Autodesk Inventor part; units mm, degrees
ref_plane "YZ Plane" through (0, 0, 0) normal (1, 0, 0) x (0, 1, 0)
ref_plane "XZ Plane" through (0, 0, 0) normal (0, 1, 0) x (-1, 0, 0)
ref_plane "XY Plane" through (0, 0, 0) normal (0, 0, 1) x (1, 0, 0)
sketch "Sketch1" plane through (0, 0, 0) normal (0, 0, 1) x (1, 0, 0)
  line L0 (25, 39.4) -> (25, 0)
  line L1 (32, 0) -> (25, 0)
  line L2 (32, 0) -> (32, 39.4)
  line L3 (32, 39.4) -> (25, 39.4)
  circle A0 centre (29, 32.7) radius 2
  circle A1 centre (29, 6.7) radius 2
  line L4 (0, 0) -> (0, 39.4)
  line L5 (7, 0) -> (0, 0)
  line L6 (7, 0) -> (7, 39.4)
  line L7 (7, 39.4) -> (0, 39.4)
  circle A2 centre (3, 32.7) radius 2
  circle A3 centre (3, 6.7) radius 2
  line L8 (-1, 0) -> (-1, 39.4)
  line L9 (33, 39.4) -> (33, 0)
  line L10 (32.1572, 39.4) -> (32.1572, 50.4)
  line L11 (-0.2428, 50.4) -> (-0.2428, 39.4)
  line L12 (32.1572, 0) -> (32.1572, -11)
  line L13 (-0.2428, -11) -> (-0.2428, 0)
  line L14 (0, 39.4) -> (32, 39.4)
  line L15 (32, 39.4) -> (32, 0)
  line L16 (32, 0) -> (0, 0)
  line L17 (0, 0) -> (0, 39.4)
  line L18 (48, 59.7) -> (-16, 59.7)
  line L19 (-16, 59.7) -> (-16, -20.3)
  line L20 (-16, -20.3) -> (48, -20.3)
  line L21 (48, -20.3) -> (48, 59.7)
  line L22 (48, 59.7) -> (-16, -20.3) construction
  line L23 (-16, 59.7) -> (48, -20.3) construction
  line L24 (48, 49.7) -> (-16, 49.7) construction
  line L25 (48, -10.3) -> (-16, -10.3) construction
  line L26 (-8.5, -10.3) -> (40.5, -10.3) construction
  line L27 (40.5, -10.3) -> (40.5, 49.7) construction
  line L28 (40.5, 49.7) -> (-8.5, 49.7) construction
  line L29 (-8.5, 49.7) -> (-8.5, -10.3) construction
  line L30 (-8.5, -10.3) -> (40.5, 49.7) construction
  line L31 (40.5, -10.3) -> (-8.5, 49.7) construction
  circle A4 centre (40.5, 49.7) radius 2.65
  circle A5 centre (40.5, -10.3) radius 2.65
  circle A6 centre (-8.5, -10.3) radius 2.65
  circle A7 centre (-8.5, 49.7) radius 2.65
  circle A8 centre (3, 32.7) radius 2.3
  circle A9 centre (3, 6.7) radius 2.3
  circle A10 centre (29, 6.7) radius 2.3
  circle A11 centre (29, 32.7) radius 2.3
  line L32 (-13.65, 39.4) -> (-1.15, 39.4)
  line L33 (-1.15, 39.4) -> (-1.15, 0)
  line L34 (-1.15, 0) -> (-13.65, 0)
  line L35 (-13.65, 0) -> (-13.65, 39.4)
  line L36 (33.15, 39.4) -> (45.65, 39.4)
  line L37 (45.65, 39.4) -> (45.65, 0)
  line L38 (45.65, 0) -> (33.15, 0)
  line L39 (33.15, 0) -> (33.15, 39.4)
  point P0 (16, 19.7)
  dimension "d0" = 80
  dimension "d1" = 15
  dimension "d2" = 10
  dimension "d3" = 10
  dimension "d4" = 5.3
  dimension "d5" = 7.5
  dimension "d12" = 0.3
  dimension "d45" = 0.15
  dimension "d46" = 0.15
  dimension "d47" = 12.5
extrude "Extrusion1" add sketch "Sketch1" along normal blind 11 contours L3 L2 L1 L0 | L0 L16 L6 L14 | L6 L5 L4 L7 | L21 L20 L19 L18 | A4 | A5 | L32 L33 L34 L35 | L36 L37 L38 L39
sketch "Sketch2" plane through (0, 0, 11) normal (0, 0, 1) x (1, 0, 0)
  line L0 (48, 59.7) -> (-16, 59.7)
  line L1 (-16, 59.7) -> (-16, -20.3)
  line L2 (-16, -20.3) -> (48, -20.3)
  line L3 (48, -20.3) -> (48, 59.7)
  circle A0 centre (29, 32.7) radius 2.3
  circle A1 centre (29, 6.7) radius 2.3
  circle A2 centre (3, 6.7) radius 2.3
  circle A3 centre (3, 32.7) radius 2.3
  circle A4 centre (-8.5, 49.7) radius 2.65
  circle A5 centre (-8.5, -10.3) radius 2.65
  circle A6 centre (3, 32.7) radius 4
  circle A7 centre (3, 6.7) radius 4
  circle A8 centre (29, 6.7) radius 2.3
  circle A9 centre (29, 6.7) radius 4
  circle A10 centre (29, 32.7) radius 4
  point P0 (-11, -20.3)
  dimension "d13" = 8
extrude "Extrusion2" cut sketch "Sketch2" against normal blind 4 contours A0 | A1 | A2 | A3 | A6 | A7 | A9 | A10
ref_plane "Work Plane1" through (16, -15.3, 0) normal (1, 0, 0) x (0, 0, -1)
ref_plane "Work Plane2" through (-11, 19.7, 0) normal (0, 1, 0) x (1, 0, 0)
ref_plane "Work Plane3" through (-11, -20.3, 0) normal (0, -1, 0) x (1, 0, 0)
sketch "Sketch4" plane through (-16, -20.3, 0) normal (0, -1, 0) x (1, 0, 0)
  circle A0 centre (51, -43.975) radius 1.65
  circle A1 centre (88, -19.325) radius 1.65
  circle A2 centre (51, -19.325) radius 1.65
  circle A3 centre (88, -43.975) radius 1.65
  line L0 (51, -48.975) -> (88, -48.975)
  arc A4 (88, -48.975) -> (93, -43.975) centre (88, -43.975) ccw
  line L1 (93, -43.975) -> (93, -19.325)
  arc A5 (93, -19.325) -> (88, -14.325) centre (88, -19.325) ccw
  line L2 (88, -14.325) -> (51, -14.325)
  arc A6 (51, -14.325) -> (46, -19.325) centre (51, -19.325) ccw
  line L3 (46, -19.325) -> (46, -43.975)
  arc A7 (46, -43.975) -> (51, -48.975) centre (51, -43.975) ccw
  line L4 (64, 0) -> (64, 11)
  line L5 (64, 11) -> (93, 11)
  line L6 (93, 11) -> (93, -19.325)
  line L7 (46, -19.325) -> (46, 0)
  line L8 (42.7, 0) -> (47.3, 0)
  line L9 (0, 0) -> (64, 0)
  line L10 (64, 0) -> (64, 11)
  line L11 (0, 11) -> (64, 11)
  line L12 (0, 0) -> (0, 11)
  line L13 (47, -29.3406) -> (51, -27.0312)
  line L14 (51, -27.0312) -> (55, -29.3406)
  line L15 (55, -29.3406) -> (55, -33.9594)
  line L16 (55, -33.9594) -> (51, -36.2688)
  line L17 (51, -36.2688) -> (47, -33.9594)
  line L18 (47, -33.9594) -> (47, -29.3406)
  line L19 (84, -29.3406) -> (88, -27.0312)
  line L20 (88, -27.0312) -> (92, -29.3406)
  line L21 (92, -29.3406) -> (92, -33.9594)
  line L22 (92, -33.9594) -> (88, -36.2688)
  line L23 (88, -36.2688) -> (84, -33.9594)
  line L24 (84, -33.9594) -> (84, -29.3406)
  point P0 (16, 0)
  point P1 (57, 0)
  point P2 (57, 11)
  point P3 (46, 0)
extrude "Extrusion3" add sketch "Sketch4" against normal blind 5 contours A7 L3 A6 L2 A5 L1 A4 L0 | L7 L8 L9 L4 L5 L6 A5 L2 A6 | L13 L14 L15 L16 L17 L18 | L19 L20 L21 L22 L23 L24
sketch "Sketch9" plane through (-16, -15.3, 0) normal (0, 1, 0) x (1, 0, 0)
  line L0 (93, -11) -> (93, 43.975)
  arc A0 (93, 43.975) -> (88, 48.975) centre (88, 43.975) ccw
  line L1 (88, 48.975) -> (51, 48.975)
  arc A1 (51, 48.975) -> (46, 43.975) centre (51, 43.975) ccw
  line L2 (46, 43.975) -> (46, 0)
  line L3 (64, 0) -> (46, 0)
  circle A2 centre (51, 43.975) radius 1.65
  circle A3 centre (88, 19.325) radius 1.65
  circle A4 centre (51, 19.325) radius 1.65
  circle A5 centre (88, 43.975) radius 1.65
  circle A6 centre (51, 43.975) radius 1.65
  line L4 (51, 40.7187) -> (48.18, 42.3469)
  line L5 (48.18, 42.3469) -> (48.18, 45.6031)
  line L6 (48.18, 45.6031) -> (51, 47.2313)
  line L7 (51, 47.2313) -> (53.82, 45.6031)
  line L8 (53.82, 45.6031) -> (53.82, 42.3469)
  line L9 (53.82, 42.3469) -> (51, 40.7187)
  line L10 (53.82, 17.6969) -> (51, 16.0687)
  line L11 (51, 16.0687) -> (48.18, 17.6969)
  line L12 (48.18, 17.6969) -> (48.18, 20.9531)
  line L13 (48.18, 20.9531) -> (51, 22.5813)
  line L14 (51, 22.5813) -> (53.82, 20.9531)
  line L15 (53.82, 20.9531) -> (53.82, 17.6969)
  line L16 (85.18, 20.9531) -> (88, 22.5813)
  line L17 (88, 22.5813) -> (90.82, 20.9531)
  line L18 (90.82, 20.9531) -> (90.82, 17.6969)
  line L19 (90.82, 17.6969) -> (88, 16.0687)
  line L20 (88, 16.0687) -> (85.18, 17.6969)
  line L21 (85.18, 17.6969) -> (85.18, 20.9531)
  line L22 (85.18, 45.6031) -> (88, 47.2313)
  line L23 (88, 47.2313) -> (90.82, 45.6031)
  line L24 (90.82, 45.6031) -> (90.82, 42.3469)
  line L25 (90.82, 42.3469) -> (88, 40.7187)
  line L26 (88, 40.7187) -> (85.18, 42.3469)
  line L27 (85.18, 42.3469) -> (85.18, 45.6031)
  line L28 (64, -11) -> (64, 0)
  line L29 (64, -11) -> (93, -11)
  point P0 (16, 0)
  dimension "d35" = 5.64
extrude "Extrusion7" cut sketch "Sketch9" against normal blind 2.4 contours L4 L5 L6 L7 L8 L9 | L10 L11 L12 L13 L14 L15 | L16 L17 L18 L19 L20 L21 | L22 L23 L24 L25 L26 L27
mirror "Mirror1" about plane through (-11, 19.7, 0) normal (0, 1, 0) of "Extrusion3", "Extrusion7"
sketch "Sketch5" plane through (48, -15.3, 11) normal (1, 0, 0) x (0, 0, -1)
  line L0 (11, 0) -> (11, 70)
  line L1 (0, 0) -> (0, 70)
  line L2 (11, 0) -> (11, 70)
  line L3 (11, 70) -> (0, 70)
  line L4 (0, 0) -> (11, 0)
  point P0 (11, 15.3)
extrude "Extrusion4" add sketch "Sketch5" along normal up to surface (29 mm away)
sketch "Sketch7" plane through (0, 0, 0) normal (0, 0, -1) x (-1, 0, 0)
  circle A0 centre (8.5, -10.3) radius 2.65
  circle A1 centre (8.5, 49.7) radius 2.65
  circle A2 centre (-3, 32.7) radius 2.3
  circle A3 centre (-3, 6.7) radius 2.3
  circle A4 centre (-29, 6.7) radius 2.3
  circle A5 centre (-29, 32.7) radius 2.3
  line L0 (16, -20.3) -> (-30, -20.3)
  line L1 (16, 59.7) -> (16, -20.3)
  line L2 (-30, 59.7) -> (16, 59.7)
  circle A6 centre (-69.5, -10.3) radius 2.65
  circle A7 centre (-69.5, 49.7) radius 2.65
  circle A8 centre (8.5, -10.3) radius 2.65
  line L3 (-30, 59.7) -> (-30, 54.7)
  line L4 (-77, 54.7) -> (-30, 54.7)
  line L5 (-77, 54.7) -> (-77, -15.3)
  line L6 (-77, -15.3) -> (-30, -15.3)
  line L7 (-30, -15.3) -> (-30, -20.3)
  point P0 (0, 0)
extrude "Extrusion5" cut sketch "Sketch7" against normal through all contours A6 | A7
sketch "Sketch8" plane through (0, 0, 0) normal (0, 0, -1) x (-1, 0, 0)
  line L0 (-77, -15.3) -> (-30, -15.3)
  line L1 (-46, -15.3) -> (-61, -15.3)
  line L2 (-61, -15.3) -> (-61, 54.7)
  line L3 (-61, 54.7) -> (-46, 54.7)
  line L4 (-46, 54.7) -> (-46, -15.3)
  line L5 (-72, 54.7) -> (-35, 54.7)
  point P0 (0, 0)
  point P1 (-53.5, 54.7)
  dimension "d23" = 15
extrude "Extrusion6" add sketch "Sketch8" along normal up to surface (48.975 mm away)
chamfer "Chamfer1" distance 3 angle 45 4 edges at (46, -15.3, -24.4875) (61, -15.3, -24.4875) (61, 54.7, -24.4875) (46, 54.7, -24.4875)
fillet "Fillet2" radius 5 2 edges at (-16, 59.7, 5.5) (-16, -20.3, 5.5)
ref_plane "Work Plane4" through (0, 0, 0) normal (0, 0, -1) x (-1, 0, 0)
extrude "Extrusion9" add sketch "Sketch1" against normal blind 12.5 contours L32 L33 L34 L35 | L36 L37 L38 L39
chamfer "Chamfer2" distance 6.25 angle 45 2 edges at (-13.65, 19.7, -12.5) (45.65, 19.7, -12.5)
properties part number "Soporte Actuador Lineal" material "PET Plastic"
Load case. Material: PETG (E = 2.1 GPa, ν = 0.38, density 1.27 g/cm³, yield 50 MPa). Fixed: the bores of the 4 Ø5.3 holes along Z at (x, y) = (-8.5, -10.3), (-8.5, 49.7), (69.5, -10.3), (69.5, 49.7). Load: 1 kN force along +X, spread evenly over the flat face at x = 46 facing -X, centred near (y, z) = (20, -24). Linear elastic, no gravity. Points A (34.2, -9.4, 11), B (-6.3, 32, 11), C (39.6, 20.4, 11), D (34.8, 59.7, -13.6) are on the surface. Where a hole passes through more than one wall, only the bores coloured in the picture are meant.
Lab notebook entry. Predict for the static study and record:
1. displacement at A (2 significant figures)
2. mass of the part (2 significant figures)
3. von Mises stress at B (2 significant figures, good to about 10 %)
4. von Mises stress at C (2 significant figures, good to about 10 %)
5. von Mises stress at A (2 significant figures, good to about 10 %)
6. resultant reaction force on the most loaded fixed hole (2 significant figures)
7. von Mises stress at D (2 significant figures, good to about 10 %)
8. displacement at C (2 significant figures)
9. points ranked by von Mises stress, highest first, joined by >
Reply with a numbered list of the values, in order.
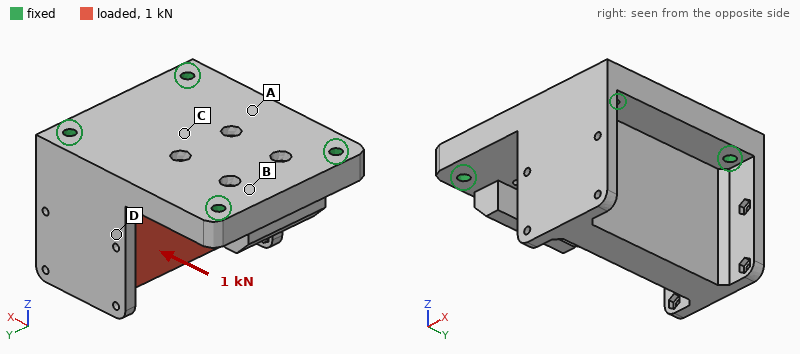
1. 0.16 mm
2. 210 g
3. 0.90 MPa
4. 3.2 MPa
5. 4.7 MPa
6. 380 N
7. 2.0 MPa
8. 0.14 mm
9. A > C > D > B
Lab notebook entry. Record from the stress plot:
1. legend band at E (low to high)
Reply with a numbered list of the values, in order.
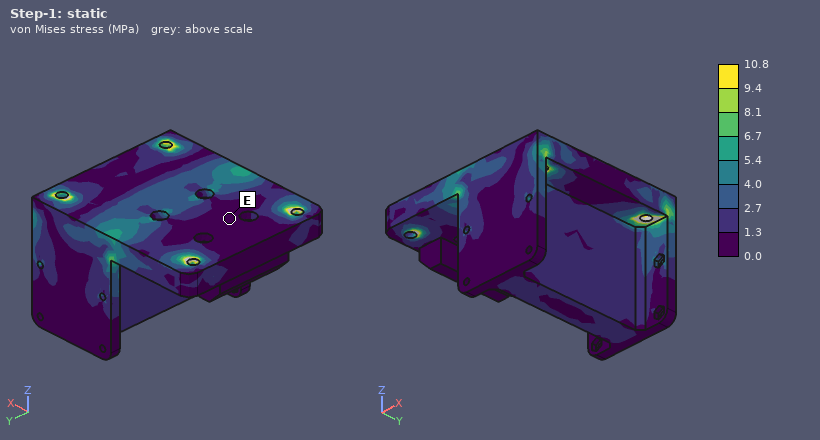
1. 0.0 to 1.3 MPa
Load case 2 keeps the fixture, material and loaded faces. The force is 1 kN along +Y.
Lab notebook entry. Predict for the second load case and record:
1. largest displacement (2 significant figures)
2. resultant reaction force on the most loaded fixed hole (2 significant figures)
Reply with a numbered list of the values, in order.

1. 0.13 mm
2. 620 N
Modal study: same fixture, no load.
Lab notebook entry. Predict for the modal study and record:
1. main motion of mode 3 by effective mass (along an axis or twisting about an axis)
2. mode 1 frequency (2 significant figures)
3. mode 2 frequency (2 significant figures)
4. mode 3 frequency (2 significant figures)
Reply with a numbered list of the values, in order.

1. along Y
2. 810 Hz
3. 1200 Hz
4. 1800 Hz
